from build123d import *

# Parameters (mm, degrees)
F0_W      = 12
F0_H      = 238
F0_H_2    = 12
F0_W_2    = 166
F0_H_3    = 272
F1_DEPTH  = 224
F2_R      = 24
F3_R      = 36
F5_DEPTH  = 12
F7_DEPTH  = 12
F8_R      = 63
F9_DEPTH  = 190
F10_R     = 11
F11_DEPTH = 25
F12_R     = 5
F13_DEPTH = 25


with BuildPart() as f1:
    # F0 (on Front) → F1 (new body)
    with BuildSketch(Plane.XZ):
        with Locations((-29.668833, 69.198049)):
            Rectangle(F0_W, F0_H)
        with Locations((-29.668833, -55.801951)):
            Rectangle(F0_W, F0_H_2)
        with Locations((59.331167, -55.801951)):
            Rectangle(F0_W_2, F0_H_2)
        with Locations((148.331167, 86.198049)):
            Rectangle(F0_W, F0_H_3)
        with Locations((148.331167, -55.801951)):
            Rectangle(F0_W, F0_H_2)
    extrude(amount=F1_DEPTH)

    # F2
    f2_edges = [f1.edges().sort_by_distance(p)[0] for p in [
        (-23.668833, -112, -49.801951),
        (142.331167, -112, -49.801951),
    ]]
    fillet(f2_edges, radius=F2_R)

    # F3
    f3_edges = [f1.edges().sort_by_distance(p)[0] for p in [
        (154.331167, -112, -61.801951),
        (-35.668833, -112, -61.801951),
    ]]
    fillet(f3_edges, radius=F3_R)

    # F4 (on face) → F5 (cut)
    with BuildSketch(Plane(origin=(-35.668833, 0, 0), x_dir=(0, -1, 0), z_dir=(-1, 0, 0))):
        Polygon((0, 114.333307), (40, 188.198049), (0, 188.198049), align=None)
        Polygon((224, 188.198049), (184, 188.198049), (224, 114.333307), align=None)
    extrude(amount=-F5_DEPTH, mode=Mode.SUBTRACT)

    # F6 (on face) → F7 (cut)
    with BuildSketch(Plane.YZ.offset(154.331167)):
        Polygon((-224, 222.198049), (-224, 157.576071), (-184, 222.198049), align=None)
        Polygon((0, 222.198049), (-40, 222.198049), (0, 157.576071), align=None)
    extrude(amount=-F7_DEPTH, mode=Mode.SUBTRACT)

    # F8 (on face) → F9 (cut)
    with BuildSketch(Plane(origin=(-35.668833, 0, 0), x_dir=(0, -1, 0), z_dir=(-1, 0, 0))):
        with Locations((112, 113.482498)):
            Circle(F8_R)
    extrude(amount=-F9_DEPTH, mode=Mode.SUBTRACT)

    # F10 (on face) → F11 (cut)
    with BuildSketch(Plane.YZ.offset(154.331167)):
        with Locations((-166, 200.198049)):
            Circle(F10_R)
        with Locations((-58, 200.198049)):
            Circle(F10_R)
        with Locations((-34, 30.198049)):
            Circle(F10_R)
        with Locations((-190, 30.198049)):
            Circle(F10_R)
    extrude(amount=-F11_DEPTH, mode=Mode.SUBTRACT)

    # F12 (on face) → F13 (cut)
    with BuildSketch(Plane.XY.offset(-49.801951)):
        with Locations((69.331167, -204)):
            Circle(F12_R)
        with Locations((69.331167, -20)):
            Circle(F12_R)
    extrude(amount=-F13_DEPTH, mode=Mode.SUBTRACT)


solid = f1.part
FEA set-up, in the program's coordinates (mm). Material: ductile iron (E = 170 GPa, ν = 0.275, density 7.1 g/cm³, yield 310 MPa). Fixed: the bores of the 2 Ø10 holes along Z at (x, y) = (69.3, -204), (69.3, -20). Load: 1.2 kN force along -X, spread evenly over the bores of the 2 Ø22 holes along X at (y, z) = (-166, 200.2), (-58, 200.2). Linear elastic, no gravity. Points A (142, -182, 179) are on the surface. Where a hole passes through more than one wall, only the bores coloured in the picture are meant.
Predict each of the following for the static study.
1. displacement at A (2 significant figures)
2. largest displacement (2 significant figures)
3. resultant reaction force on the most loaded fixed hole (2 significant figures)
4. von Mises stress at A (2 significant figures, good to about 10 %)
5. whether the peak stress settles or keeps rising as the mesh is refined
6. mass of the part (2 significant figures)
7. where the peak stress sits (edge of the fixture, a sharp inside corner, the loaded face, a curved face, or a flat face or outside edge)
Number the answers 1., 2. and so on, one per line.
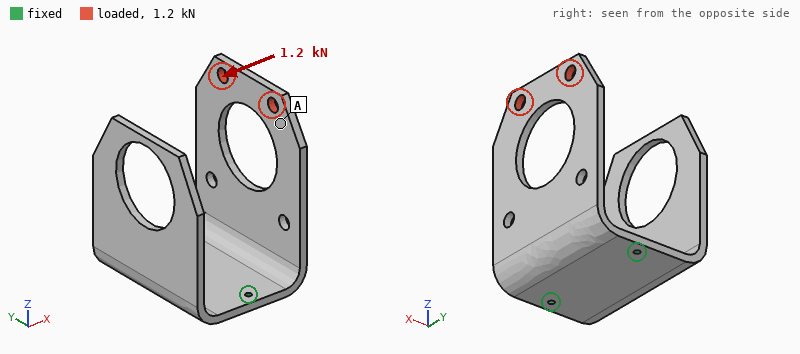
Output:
1. 2.3 mm
2. 3.0 mm
3. 620 N
4. 12 MPa
5. keeps rising
6. 10 kg
7. edge of the fixture
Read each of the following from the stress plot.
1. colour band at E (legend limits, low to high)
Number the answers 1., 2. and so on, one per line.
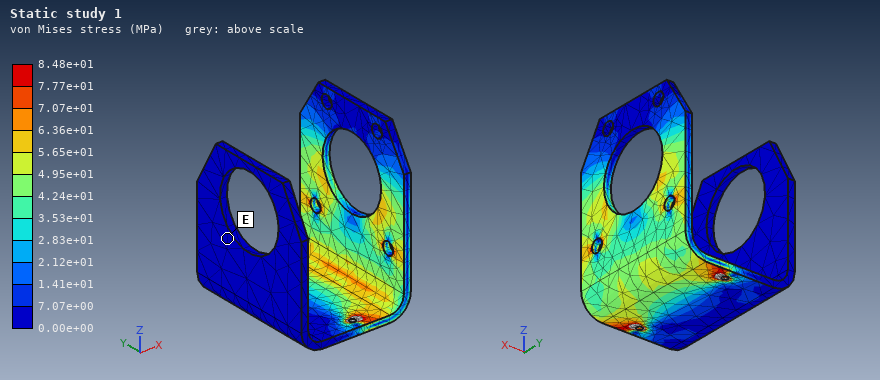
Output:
1. 0.00e+00 to 7.07e+00 MPa
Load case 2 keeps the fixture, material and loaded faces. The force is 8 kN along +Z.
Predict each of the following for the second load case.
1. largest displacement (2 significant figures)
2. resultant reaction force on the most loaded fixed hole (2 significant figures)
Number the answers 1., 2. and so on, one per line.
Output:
1. 1.8 mm
2. 4.0 kN
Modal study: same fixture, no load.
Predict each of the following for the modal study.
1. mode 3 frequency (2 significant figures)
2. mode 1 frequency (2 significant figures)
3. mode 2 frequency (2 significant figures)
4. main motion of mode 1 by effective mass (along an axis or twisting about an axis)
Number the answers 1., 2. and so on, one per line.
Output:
1. 260 Hz
2. 99 Hz
3. 130 Hz
4. along X
